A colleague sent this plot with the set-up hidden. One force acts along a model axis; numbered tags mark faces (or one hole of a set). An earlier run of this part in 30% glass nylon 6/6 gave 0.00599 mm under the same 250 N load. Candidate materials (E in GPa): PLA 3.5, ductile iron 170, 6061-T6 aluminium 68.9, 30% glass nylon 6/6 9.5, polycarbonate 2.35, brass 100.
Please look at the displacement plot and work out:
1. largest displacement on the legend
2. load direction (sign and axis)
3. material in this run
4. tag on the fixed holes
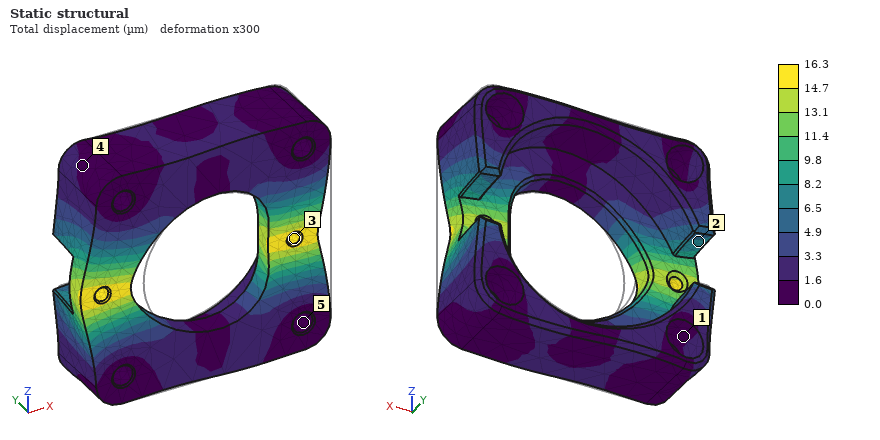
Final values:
16.3 µm
-X
PLA
5
